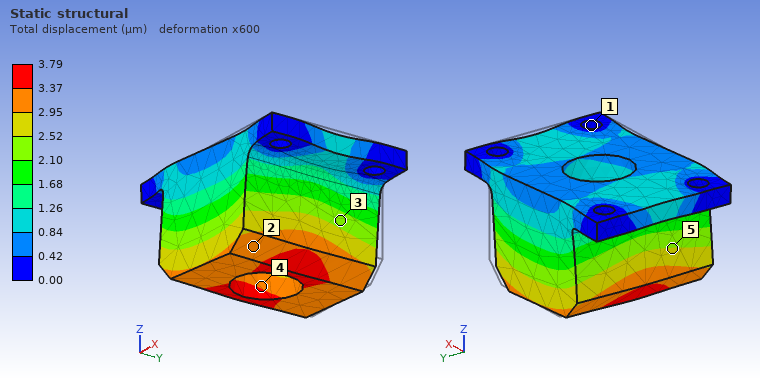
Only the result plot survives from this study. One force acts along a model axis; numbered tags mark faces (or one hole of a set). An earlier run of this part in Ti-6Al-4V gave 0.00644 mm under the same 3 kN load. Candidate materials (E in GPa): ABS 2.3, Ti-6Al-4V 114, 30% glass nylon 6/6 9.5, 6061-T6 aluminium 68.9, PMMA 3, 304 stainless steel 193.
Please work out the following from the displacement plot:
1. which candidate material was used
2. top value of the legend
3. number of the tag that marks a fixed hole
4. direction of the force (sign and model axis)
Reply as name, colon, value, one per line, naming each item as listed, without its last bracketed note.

which candidate material was used: 304 stainless steel
top value of the legend: 3.79 µm
number of the tag that marks a fixed hole: 1
direction of the force: -X
